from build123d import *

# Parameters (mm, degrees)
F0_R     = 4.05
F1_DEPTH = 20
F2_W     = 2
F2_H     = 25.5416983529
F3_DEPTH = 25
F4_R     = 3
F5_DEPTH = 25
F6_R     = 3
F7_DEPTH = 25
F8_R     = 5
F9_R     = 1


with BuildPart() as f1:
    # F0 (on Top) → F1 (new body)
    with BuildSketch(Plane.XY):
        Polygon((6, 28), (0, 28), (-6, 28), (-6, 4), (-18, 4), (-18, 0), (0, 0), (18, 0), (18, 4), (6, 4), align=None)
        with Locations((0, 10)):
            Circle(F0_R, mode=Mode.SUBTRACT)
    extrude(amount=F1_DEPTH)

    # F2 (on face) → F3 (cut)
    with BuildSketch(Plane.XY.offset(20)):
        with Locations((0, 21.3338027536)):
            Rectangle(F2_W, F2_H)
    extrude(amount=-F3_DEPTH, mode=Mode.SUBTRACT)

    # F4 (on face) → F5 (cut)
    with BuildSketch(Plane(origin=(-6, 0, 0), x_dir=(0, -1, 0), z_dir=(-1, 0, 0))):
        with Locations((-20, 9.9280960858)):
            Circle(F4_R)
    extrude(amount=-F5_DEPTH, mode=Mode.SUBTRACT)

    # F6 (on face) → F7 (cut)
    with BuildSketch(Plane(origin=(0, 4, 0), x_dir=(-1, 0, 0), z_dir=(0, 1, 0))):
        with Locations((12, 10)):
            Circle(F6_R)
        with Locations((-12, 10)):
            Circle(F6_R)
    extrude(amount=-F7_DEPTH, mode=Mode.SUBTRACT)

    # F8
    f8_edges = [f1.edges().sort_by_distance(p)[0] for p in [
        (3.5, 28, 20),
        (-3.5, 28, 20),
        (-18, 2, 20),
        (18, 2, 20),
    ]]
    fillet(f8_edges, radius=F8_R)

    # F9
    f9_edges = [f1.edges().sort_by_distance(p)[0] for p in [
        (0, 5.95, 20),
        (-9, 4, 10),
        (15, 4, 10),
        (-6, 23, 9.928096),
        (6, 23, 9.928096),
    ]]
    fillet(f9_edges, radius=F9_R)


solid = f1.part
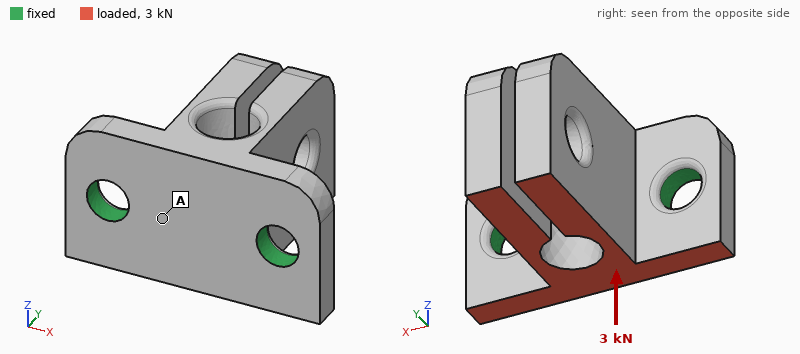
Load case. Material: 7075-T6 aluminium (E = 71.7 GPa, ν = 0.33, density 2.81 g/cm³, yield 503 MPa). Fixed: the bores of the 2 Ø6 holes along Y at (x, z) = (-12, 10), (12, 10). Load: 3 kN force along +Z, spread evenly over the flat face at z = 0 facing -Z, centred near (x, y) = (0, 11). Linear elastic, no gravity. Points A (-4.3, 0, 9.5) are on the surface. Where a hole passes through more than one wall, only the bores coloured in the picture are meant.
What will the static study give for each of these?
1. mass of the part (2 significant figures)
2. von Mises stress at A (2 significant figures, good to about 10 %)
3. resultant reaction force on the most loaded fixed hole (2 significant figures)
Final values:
18 g
42 MPa
1.5 kN
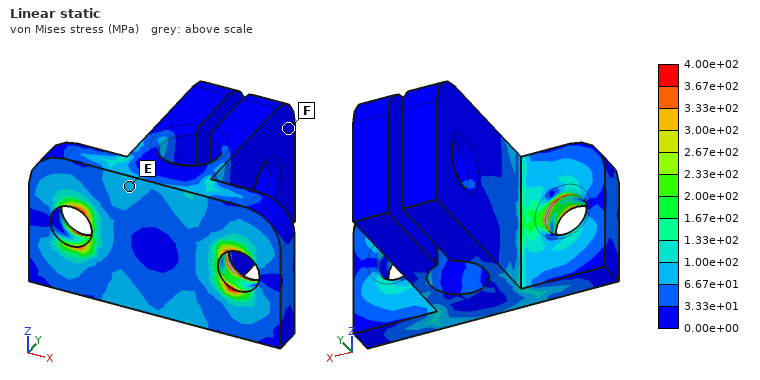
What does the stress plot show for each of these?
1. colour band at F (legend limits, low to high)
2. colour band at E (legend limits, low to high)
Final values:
0.00e+00 to 3.33e+01 MPa
6.67e+01 to 1.00e+02 MPa
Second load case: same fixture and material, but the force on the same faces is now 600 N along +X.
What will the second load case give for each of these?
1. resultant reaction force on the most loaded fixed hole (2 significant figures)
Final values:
480 N
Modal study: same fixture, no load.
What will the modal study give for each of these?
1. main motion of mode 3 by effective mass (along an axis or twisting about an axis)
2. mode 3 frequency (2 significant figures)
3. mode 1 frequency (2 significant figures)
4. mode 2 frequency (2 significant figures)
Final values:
along Z
5500 Hz
2900 Hz
3000 Hz
